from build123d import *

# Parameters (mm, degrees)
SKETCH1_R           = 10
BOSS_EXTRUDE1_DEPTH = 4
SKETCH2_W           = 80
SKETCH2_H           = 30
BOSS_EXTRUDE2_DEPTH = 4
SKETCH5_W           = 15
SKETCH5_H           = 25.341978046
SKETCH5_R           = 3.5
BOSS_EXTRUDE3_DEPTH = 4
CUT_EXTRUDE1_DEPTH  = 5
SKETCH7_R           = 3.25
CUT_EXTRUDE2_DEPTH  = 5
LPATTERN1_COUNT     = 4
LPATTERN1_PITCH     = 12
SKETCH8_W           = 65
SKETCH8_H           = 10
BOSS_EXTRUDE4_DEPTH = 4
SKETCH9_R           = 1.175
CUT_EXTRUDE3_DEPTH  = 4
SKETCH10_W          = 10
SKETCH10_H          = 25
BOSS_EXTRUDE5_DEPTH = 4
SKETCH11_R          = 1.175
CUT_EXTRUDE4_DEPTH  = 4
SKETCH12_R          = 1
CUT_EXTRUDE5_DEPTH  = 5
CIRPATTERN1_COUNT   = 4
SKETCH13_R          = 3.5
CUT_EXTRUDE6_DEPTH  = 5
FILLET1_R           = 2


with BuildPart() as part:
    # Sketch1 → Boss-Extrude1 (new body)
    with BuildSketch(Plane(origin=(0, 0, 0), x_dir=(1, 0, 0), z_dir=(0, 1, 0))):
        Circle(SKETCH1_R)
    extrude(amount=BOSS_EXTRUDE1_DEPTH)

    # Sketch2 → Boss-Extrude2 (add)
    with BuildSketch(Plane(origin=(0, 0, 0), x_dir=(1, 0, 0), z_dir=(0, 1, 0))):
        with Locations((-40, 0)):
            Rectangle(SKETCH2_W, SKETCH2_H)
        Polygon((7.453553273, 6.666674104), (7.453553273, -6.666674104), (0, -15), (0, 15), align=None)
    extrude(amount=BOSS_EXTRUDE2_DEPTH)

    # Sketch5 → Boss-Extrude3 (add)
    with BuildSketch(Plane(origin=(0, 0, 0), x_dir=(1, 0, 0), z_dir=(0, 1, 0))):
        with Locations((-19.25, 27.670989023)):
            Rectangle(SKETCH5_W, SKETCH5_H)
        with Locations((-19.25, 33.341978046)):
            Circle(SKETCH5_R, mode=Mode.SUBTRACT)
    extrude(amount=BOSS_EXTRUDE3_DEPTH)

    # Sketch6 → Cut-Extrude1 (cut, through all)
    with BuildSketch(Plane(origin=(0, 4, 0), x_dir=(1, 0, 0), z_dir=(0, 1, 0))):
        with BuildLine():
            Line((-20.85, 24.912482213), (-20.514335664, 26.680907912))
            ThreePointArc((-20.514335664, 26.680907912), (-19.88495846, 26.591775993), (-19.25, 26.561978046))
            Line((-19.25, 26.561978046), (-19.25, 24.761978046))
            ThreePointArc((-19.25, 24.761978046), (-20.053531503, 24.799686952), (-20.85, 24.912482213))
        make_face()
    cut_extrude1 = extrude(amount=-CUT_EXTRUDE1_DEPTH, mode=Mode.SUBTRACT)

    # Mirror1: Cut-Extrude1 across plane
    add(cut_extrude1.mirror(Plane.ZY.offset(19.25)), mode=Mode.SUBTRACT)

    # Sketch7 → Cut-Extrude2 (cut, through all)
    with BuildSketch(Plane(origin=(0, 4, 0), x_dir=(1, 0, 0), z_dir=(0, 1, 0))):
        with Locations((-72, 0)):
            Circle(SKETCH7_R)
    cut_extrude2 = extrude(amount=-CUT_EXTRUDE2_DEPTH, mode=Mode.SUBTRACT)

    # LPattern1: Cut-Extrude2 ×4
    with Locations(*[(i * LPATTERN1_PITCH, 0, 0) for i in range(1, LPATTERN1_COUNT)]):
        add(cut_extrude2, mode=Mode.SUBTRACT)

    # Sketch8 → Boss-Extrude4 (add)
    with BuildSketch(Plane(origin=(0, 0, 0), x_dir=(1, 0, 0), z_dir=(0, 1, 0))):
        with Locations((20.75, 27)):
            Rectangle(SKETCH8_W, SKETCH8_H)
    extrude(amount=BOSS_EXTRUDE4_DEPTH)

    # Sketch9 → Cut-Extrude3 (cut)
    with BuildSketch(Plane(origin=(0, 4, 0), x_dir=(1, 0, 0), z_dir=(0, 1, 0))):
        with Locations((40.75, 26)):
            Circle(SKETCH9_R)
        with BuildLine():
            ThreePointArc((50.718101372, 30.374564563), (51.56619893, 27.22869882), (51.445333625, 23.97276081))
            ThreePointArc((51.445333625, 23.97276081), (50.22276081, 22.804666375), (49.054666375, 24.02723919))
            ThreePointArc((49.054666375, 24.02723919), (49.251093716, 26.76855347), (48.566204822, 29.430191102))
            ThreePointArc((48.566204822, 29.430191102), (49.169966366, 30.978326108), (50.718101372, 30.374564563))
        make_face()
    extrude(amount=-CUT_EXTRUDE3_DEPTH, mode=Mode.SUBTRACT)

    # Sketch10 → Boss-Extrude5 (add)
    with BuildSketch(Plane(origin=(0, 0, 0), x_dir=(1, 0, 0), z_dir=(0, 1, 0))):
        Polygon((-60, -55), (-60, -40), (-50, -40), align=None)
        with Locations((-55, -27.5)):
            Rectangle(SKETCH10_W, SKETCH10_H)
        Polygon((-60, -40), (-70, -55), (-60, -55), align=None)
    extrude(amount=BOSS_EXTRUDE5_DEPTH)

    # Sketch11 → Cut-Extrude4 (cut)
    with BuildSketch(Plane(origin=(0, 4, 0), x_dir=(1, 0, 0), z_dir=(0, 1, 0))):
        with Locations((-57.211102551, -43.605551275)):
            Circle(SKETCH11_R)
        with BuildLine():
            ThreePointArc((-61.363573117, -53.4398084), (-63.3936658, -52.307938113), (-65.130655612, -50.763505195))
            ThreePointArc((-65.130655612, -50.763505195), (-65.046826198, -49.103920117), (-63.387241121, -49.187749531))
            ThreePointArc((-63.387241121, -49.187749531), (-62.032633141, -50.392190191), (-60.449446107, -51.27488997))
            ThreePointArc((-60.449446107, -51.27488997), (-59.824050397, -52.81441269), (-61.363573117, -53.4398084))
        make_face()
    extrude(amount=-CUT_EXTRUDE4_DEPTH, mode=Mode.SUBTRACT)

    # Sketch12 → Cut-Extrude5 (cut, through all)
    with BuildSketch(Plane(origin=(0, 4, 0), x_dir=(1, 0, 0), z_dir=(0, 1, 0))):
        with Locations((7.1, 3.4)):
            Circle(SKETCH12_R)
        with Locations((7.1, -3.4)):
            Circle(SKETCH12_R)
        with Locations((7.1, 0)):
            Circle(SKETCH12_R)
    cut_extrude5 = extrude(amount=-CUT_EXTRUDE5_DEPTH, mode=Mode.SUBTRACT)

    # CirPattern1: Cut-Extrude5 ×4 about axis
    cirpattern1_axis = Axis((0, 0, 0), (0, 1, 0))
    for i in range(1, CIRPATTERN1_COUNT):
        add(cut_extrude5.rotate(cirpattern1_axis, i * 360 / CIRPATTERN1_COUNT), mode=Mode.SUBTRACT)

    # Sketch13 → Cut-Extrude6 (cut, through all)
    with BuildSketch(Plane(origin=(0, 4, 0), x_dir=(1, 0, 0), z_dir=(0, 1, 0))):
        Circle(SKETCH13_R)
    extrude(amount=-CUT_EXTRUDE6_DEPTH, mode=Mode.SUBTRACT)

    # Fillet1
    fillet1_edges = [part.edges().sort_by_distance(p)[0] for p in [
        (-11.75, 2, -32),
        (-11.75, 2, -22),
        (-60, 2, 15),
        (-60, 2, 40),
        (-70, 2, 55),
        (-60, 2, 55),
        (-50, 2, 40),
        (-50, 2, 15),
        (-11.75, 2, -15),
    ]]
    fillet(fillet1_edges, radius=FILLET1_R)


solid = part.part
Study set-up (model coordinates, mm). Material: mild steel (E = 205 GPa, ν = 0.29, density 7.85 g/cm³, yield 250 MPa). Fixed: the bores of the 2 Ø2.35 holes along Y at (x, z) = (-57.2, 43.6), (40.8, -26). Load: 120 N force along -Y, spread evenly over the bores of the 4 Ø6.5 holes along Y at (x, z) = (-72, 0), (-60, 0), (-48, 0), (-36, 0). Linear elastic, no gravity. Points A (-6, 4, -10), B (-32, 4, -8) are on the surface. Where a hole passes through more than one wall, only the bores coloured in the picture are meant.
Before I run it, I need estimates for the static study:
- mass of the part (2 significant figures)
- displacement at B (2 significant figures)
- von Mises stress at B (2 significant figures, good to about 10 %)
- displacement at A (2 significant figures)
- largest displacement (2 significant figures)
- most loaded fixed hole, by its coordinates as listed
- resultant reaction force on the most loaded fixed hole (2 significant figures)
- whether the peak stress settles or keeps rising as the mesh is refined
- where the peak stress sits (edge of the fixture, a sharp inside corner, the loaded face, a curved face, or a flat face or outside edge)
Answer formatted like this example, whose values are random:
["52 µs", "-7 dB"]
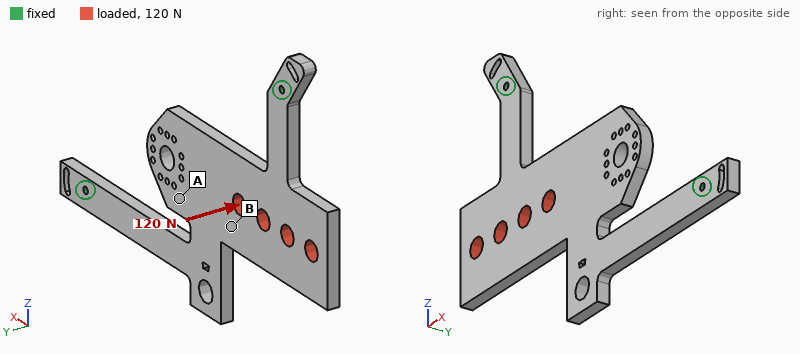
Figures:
["120 g", "0.12 mm", "17 MPa", "0.050 mm", "0.28 mm", "(-57.2, 43.6)", "96 N", "keeps rising", "edge of the fixture"]
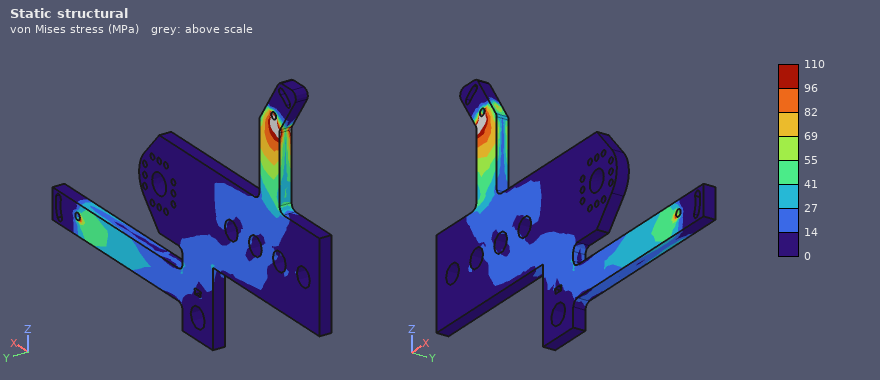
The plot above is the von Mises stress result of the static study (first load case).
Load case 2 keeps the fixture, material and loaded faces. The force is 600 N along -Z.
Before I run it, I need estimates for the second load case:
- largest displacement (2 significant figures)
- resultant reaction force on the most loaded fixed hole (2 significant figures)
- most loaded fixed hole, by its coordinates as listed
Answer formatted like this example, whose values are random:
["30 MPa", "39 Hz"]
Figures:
["4.6 µm", "600 N", "(-57.2, 43.6)"]
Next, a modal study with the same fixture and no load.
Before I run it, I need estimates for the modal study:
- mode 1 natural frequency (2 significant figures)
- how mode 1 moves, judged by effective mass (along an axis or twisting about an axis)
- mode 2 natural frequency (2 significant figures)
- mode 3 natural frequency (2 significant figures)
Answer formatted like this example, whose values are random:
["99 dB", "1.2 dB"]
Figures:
["550 Hz", "along Y", "820 Hz", "1700 Hz"]
